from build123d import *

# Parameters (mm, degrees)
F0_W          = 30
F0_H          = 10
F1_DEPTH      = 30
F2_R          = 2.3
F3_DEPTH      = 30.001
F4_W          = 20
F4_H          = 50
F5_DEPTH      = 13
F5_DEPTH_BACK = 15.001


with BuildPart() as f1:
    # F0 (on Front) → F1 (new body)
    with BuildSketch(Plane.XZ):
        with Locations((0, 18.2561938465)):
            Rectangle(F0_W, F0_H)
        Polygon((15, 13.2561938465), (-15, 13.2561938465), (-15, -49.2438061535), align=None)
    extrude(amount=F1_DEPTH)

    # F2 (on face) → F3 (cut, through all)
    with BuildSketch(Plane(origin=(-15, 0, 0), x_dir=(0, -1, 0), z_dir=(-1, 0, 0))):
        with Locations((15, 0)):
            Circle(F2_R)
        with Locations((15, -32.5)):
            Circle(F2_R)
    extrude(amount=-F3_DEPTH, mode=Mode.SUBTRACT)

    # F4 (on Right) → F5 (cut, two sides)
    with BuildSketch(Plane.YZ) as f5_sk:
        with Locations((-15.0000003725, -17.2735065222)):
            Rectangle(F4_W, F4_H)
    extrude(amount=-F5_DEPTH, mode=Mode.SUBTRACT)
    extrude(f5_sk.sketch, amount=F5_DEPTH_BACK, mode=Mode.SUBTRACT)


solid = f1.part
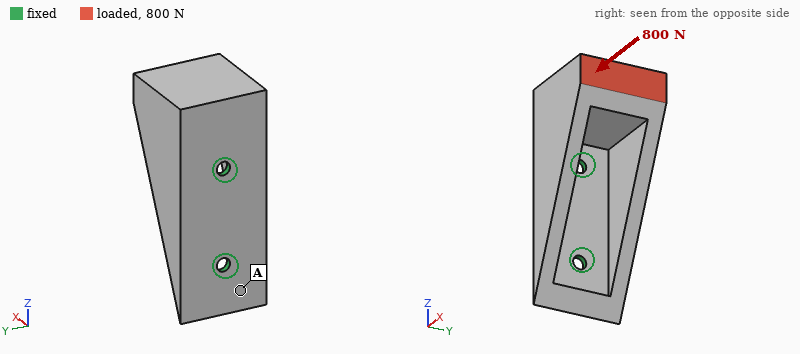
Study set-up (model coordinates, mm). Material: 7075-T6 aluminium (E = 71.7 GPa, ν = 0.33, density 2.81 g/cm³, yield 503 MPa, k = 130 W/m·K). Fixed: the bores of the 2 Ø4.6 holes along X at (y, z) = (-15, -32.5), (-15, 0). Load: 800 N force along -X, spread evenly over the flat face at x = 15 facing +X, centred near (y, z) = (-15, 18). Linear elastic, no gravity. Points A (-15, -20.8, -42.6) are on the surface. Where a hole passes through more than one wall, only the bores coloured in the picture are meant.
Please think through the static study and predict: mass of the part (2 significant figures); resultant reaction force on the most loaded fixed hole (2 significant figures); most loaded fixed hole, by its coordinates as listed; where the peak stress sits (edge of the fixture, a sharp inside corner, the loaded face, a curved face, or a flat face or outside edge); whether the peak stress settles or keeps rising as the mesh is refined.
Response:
67 g
1.2 kN
(-15, 0)
edge of the fixture
keeps rising
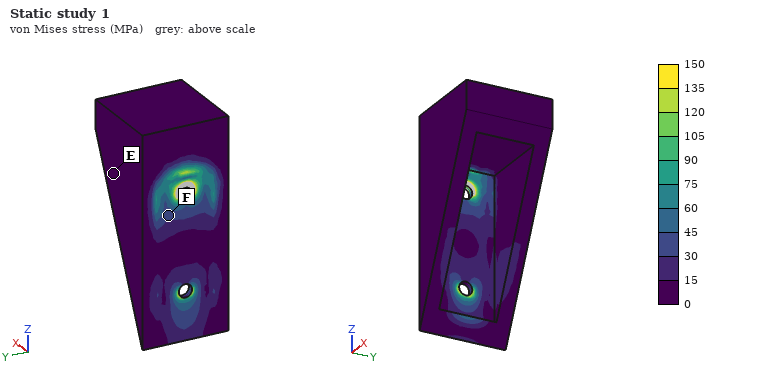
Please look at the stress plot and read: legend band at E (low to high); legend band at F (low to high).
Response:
0 to 15 MPa
30 to 45 MPa
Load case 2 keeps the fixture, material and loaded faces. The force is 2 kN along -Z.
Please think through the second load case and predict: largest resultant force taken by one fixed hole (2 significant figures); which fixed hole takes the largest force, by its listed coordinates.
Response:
2.3 kN
(-15, -32.5)
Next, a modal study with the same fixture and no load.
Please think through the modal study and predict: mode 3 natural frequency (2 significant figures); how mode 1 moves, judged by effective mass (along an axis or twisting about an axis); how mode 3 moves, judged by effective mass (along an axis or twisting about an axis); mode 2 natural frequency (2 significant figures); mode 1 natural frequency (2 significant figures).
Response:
5000 Hz
along Y
along X
2400 Hz
1200 Hz
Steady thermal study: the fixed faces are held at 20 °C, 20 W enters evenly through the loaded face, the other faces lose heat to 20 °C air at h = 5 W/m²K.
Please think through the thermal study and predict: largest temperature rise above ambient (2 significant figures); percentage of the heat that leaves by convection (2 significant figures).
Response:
26 K
3.1 %
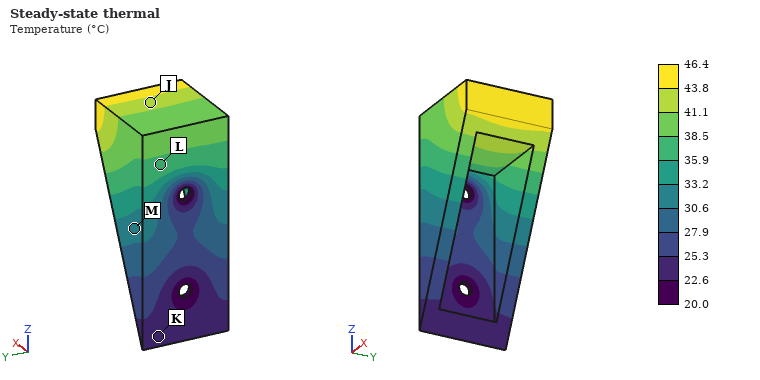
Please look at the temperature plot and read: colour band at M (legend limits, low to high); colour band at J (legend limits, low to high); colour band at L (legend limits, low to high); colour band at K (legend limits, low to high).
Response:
30.6 to 33.2 °C
41.1 to 43.8 °C
35.9 to 38.5 °C
22.6 to 25.3 °C
